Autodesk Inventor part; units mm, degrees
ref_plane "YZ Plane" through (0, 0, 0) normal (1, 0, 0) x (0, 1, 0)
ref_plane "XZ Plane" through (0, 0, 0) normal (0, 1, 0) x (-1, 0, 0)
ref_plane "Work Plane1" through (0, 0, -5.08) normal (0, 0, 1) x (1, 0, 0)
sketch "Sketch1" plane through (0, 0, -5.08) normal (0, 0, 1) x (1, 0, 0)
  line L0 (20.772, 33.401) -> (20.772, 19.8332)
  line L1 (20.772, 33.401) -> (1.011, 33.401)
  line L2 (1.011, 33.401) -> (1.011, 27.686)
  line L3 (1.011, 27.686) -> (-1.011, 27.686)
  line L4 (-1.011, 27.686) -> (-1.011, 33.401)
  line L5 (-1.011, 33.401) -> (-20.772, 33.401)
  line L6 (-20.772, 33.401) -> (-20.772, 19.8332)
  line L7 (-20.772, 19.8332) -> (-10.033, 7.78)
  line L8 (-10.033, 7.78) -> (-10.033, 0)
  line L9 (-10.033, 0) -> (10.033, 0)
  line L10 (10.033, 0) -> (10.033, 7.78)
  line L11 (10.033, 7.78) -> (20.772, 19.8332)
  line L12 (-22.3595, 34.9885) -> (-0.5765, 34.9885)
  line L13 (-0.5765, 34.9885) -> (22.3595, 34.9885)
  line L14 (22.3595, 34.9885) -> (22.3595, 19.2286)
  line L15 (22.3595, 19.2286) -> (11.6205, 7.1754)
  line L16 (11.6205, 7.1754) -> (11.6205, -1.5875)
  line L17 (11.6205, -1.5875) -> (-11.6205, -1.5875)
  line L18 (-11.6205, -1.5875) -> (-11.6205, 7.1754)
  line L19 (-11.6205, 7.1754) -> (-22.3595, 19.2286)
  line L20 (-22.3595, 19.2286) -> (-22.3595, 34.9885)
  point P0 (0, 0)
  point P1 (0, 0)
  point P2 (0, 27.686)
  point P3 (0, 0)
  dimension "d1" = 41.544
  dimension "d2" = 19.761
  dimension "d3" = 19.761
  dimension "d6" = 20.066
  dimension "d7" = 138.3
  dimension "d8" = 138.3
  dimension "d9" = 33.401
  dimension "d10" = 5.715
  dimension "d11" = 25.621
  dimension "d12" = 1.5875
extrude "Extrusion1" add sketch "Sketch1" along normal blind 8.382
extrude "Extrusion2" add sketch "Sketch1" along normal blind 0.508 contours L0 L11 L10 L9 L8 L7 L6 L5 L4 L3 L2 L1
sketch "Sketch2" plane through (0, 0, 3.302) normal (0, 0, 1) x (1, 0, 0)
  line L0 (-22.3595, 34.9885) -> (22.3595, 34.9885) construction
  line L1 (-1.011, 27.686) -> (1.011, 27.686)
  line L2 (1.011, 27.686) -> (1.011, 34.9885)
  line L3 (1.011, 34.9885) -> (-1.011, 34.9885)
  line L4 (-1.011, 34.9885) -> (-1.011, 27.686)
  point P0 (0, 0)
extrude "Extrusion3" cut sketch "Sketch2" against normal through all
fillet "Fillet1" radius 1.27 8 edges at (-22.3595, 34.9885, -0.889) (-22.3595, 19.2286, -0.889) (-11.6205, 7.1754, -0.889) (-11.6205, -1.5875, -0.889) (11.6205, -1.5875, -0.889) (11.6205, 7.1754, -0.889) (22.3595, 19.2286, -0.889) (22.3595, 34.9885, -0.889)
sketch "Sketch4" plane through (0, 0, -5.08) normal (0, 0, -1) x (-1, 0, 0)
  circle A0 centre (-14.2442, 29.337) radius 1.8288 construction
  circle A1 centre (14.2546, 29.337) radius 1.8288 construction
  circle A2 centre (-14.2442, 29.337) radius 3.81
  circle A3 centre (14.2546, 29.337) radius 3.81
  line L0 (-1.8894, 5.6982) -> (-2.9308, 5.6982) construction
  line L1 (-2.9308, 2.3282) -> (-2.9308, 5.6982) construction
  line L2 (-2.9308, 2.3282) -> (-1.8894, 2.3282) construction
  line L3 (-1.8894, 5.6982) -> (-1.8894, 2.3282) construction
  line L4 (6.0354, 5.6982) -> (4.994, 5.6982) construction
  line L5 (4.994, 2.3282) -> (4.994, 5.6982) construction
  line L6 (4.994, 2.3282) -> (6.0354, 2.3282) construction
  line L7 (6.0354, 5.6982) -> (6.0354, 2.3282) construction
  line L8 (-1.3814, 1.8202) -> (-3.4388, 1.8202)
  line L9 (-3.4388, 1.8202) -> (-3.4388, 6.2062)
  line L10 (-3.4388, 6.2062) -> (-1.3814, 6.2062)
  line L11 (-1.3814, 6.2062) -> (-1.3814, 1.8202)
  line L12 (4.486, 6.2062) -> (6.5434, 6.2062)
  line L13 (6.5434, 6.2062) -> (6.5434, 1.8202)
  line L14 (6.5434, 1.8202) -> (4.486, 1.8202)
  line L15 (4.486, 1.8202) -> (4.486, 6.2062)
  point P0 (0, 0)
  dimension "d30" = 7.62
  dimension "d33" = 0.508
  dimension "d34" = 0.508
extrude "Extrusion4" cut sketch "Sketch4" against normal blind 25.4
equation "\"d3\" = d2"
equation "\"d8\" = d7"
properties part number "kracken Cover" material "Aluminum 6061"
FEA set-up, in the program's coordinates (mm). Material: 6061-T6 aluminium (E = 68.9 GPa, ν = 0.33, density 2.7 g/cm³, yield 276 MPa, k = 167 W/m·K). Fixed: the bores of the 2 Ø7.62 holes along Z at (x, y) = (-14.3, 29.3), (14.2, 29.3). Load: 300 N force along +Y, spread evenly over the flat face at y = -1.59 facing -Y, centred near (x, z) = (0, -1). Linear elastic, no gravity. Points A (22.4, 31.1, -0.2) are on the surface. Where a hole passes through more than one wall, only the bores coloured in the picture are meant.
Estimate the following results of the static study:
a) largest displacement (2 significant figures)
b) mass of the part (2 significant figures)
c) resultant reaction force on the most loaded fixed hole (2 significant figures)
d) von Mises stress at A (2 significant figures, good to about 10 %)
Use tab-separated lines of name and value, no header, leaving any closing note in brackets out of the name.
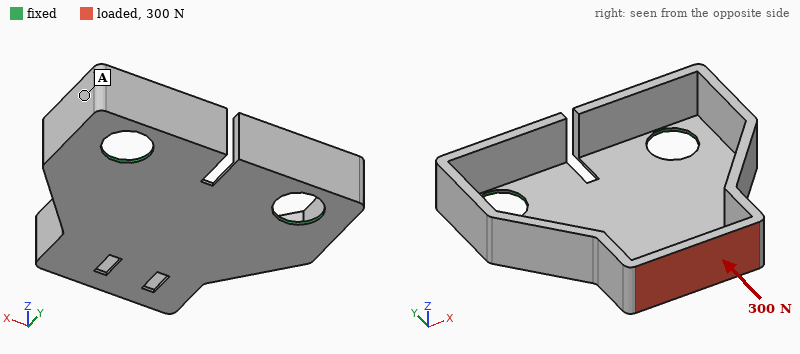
largest displacement	0.45 mm
mass of the part	6.4 g
resultant reaction force on the most loaded fixed hole	160 N
von Mises stress at A	29 MPa
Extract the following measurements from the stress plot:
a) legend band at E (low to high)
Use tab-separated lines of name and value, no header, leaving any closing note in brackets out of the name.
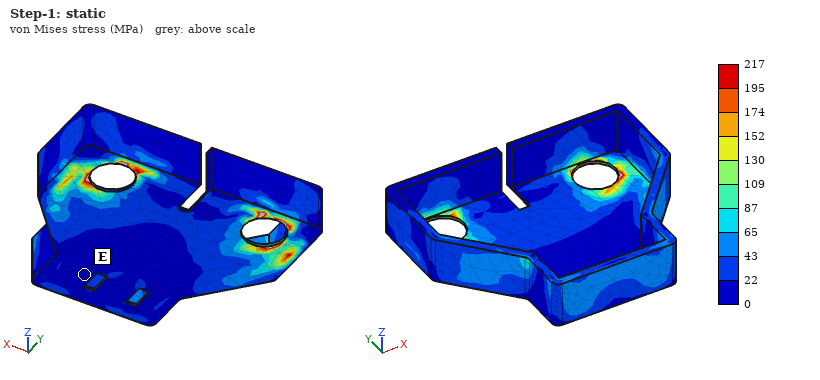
legend band at E	0 to 22 MPa
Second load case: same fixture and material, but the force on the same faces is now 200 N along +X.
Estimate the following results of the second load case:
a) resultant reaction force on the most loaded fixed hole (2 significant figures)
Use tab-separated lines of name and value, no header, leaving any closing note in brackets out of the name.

resultant reaction force on the most loaded fixed hole	200 N
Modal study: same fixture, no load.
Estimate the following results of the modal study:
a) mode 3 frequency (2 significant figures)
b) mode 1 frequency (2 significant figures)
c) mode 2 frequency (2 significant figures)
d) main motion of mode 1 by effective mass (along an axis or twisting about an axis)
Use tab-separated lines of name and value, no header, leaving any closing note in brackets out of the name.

mode 3 frequency	4900 Hz
mode 1 frequency	1200 Hz
mode 2 frequency	3100 Hz
main motion of mode 1 by effective mass	along Z
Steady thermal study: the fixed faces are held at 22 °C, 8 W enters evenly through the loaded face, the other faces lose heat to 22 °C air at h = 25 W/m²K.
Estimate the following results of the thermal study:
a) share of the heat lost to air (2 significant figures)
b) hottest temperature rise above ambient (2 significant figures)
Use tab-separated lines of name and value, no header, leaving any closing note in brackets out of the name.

share of the heat lost to air	18 %
hottest temperature rise above ambient	41 K
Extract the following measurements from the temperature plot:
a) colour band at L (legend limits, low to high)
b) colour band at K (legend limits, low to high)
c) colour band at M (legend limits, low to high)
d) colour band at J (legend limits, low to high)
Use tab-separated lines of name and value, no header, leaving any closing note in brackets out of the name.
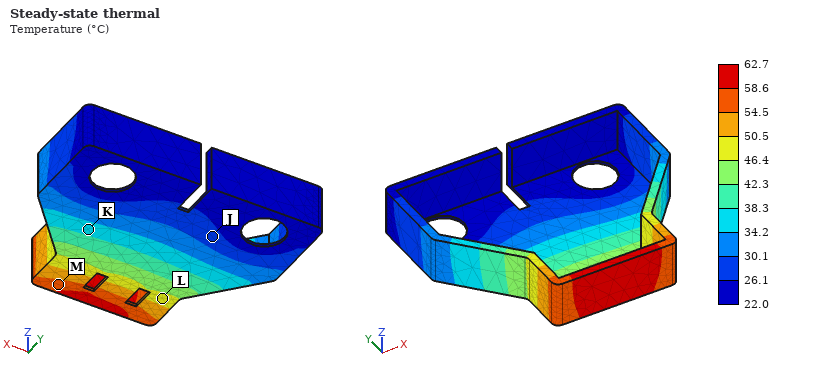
colour band at L	46.4 to 50.5 °C
colour band at K	34.2 to 38.3 °C
colour band at M	54.5 to 58.6 °C
colour band at J	26.1 to 30.1 °C
